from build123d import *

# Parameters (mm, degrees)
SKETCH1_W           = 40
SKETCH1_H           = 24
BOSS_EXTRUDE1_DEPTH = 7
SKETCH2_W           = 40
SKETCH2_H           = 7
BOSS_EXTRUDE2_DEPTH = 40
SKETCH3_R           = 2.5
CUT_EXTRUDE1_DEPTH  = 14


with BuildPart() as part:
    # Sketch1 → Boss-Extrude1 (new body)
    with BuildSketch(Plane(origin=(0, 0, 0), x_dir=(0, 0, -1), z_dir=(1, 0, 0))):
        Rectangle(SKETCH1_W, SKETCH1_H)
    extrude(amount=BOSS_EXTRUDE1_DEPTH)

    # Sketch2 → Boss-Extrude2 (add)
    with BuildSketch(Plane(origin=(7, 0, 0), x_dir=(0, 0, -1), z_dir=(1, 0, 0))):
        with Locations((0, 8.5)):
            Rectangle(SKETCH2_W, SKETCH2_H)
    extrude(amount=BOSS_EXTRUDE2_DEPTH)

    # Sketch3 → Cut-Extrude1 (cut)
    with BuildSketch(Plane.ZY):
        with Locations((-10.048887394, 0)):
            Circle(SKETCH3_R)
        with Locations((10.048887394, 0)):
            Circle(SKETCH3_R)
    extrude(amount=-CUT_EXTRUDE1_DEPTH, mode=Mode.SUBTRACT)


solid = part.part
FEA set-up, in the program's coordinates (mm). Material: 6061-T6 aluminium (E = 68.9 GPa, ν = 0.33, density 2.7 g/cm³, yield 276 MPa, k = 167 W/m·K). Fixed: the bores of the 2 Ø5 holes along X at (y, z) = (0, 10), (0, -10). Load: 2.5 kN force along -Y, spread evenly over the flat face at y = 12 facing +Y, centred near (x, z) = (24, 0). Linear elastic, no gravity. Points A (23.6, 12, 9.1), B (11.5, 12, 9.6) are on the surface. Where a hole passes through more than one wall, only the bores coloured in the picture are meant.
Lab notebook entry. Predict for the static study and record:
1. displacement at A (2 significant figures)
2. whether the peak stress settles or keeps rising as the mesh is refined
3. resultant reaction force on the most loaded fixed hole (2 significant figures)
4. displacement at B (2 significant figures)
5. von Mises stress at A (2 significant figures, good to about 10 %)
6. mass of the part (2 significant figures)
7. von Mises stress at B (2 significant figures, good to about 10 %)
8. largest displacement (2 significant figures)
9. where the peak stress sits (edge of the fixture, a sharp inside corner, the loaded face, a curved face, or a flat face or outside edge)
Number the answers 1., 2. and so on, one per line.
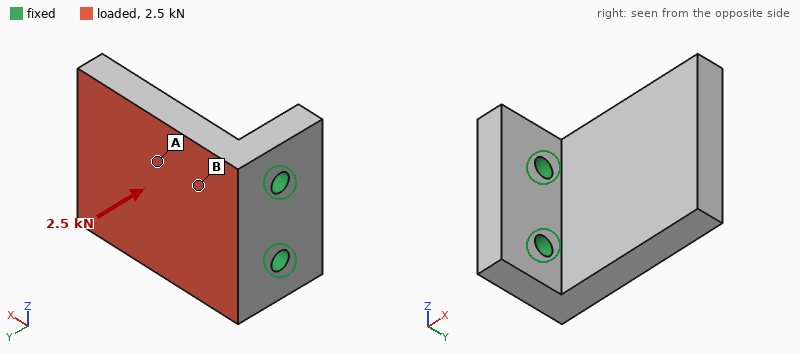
1. 0.18 mm
2. keeps rising
3. 1.3 kN
4. 0.072 mm
5. 43 MPa
6. 48 g
7. 97 MPa
8. 0.46 mm
9. edge of the fixture
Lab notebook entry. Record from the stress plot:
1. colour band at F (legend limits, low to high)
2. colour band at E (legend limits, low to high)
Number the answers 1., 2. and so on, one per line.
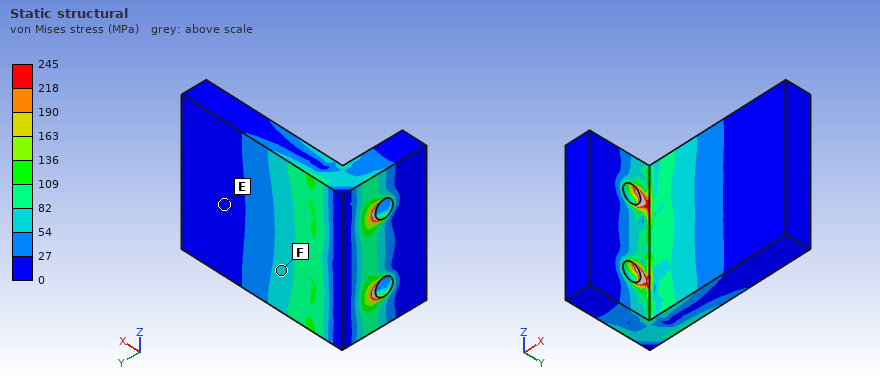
1. 54 to 82 MPa
2. 0 to 27 MPa
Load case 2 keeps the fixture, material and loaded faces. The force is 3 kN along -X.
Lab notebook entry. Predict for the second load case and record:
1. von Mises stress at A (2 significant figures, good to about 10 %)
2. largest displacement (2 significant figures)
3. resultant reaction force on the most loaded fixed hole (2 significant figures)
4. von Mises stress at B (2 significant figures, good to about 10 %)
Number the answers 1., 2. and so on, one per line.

1. 21 MPa
2. 0.18 mm
3. 1.5 kN
4. 32 MPa
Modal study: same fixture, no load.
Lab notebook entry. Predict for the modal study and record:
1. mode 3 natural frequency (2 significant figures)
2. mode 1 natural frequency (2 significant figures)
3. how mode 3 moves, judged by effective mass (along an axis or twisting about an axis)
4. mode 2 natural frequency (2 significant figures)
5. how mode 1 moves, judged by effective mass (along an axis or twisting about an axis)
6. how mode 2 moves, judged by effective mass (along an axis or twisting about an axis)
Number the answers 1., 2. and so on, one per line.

1. 7500 Hz
2. 2400 Hz
3. along Z
4. 5900 Hz
5. along Y
6. along Z
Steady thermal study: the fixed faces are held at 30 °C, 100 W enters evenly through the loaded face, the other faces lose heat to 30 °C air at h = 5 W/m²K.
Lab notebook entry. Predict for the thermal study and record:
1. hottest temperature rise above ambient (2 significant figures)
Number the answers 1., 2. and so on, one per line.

1. 56 K
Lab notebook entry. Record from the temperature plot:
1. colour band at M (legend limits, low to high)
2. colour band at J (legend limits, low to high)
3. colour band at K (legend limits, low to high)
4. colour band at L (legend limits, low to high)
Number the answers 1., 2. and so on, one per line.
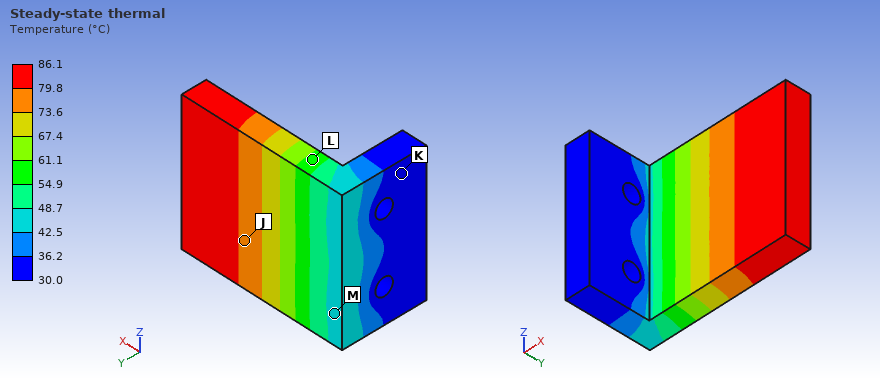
1. 42.5 to 48.7 °C
2. 73.6 to 79.8 °C
3. 30.0 to 36.2 °C
4. 54.9 to 61.1 °C
